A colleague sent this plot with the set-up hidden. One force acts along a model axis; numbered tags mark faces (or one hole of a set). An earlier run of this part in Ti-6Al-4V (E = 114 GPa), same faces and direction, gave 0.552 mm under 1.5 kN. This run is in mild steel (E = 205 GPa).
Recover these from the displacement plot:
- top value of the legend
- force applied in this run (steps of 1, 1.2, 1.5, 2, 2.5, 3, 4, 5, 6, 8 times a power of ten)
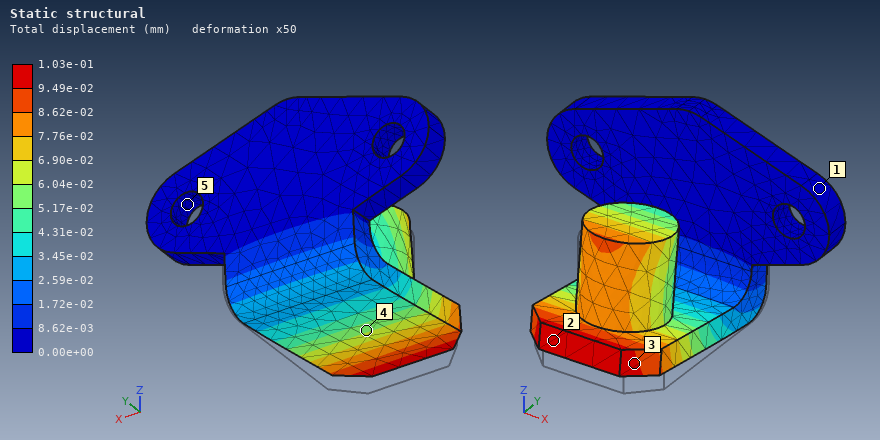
1.03e-01 mm
500 N
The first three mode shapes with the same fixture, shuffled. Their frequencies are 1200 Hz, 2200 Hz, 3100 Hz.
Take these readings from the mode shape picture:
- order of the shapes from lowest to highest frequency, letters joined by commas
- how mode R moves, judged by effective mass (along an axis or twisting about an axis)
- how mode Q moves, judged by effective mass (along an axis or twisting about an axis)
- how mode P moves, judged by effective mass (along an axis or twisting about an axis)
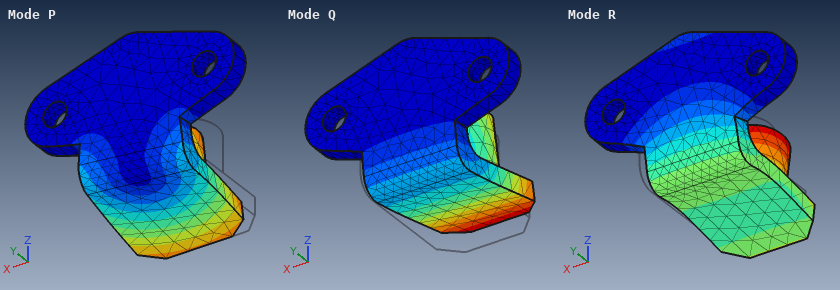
Q, P, R
along Y
along Z
along X
